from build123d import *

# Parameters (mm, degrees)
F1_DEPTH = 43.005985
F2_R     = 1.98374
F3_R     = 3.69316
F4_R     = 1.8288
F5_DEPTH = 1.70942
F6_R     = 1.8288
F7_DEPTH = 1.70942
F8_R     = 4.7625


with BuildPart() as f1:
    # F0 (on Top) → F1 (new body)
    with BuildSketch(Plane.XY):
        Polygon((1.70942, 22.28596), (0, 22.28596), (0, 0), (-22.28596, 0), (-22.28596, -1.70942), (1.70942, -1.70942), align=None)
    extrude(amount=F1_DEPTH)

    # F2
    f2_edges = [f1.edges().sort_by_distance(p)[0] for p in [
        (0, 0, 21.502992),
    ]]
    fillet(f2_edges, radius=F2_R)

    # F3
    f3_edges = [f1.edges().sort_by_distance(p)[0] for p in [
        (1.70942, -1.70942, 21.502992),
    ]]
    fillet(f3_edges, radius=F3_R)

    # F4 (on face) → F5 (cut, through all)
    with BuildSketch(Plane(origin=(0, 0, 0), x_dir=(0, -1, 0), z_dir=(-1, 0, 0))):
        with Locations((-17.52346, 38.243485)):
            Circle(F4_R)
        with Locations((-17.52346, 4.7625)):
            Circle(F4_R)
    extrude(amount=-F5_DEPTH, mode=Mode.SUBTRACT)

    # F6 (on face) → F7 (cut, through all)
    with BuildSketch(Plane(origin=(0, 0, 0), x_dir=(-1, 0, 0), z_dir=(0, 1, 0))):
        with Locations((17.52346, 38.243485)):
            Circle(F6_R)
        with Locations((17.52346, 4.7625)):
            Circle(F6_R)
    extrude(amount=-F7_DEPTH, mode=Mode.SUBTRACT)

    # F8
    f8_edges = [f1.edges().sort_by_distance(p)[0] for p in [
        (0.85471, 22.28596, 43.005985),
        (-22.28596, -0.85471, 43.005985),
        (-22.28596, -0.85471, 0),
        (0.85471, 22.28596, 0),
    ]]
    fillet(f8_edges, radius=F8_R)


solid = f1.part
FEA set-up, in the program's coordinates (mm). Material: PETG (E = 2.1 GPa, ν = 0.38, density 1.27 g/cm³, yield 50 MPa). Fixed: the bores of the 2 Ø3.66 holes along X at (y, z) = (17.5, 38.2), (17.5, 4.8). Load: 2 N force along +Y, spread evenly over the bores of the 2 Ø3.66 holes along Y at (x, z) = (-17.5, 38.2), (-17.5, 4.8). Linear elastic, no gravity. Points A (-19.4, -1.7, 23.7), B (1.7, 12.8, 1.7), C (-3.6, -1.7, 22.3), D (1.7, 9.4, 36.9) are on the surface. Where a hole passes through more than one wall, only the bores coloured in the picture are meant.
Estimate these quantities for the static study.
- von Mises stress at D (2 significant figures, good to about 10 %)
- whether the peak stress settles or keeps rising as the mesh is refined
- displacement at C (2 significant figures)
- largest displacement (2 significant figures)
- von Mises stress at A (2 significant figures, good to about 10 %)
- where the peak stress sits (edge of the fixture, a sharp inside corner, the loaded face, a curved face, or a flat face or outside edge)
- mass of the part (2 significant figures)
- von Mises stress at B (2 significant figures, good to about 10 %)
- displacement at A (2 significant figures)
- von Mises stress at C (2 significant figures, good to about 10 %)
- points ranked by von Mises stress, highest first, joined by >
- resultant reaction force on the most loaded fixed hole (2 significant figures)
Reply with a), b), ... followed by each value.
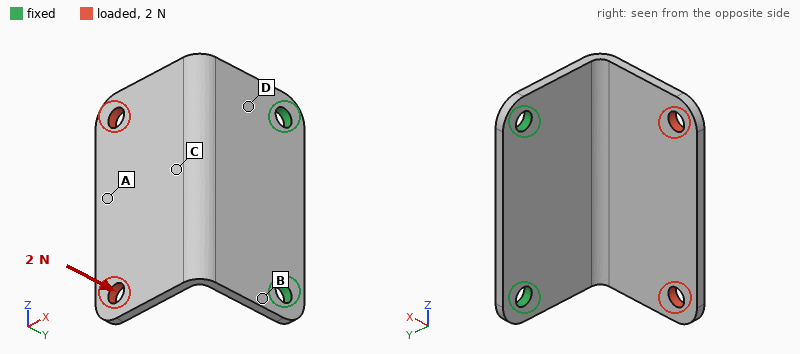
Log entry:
a) 1.7 MPa
b) keeps rising
c) 0.20 mm
d) 0.56 mm
e) 0.48 MPa
f) edge of the fixture
g) 4.1 g
h) 2.3 MPa
i) 0.47 mm
j) 1.2 MPa
k) B > D > C > A
l) 1.1 N
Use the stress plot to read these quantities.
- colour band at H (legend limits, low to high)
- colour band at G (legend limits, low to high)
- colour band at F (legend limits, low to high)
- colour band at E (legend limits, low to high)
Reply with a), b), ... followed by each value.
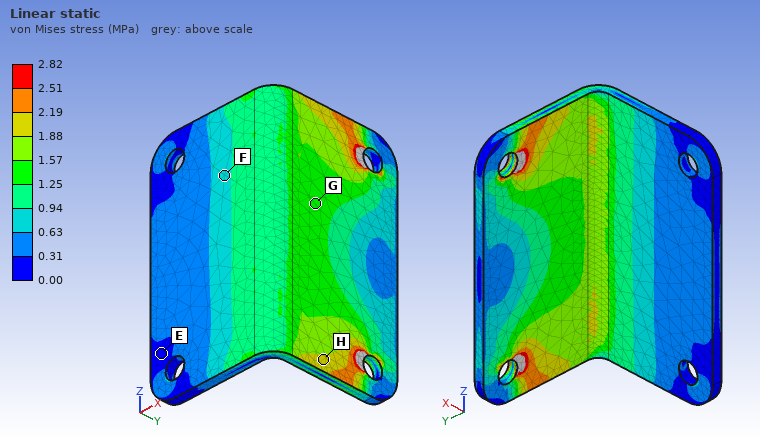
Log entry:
a) 1.88 to 2.19 MPa
b) 1.25 to 1.57 MPa
c) 0.63 to 0.94 MPa
d) 0.00 to 0.31 MPa
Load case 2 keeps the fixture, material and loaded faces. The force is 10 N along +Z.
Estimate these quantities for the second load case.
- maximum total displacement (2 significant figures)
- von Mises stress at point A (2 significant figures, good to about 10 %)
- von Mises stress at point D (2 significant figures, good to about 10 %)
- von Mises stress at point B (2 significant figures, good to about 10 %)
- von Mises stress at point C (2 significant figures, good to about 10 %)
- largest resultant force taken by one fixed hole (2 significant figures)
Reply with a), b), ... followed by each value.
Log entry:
a) 0.61 mm
b) 0.77 MPa
c) 3.5 MPa
d) 5.9 MPa
e) 1.7 MPa
f) 9.1 N
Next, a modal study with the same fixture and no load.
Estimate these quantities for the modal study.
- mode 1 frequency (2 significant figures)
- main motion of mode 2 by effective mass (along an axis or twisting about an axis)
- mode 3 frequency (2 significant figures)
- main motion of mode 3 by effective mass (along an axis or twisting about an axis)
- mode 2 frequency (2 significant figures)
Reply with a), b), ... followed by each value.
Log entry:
a) 280 Hz
b) along Z
c) 800 Hz
d) along X
e) 550 Hz
